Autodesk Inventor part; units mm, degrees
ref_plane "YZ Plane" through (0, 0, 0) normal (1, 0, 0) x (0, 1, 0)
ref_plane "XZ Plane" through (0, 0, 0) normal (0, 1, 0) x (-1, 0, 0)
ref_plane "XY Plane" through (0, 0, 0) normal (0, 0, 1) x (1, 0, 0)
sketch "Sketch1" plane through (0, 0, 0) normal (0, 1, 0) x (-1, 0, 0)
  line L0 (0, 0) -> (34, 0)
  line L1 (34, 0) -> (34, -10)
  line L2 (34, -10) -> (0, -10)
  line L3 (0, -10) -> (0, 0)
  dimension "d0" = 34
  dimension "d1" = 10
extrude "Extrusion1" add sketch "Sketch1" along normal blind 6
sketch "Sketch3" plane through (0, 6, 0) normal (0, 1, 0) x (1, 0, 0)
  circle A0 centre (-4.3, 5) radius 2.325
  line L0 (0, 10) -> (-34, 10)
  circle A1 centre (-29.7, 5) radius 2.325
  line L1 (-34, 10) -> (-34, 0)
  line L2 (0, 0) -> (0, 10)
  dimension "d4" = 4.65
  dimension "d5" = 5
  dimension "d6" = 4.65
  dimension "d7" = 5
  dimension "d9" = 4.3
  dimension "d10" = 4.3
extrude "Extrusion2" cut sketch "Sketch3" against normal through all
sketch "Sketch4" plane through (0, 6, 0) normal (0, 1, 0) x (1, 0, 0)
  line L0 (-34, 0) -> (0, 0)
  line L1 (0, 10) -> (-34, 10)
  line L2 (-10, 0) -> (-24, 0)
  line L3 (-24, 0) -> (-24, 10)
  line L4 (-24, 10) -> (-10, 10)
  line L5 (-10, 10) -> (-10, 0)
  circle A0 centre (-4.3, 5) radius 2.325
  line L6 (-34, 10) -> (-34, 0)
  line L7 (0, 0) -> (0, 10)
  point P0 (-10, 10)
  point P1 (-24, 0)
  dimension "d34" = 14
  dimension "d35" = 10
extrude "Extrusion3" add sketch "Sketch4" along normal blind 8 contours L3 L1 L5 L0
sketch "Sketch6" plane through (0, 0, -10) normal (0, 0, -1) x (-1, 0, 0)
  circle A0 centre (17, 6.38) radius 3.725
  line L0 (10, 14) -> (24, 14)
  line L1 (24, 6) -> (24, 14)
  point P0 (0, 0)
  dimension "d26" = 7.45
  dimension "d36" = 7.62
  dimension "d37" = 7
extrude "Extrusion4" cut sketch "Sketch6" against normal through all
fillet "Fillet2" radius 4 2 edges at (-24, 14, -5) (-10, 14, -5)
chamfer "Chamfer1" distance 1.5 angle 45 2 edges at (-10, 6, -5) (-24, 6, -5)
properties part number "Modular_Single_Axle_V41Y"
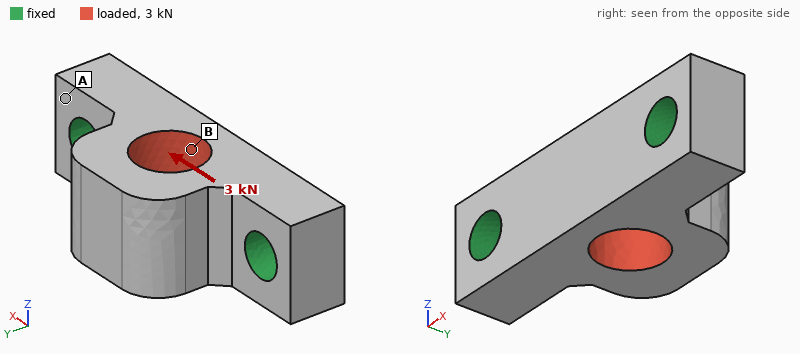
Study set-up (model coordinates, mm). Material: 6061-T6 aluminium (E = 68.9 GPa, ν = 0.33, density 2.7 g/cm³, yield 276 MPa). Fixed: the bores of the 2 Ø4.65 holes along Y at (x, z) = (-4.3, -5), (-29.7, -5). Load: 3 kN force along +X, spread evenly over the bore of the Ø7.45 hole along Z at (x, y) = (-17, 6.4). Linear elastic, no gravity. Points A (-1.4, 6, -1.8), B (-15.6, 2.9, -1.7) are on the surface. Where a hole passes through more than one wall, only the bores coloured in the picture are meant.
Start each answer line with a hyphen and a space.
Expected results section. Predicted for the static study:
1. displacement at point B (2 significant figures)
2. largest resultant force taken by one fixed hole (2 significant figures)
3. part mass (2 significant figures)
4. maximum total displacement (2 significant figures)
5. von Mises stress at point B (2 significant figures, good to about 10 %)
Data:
- 2.5 µm
- 1.6 kN
- 6.7 g
- 9.0 µm
- 24 MPa
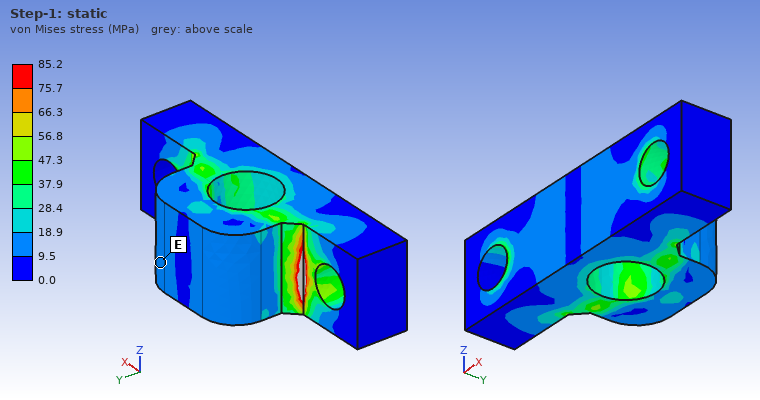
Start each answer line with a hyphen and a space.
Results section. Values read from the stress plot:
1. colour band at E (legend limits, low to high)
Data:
- 9.5 to 18.9 MPa
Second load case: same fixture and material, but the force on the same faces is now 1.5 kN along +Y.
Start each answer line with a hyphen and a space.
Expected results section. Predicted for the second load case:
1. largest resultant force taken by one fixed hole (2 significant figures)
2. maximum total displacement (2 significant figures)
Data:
- 750 N
- 8.1 µm
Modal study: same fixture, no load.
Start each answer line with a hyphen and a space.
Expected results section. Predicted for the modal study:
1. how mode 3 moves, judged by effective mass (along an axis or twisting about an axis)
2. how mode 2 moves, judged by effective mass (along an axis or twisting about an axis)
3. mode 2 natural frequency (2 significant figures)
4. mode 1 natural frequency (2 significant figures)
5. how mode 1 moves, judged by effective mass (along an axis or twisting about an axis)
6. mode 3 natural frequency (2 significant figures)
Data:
- along X
- along Y
- 42 kHz
- 23 kHz
- along Z
- 48 kHz
